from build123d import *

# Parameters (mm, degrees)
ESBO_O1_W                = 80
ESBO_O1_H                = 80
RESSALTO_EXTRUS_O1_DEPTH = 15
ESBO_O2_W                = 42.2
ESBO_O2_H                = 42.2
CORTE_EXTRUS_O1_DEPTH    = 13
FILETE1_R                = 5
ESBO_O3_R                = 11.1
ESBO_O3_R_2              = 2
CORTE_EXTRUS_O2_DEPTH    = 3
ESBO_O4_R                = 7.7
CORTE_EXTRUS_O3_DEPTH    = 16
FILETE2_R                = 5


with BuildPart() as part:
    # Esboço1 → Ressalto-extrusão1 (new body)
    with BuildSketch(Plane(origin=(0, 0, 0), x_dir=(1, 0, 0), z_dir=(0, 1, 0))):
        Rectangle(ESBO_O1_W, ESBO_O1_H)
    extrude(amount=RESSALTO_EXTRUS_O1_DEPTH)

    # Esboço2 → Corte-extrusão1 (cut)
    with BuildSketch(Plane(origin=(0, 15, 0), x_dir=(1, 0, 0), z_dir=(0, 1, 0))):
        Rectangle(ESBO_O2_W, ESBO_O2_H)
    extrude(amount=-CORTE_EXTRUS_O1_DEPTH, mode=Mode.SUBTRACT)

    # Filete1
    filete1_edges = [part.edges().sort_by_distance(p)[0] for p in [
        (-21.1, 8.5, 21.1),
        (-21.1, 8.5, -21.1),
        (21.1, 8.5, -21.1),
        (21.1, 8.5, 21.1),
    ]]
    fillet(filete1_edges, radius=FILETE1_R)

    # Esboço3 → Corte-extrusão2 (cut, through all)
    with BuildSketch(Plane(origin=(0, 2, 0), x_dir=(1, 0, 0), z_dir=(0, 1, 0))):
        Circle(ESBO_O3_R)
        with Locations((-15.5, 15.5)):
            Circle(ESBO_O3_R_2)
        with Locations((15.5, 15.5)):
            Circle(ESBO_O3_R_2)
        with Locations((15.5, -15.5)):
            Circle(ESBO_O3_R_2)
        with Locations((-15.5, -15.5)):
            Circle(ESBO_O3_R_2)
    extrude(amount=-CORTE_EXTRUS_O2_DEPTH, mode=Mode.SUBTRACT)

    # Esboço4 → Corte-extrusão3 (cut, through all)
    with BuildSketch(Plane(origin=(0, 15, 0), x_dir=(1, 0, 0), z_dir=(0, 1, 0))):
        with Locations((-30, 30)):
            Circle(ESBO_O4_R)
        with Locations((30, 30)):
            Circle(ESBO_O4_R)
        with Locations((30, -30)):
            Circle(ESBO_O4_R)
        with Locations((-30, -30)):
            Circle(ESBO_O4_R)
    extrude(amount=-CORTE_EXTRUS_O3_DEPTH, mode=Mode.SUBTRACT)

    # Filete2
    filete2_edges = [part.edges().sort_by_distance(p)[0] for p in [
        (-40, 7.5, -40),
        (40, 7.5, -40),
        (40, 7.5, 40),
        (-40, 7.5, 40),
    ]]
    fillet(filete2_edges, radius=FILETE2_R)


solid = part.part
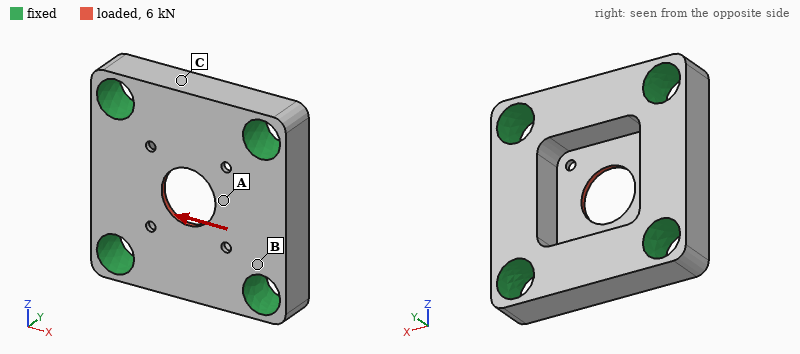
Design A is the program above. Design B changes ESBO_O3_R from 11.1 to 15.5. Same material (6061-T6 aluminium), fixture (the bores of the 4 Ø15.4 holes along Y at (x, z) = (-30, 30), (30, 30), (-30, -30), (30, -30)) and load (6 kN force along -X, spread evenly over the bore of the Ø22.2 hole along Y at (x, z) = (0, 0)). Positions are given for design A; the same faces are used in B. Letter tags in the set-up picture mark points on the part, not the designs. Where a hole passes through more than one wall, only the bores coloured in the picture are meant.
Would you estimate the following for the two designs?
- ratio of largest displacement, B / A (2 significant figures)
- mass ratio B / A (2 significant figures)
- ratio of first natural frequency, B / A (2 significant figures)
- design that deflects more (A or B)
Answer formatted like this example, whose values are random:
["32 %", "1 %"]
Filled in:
["0.82", "0.99", "1.6", "A"]
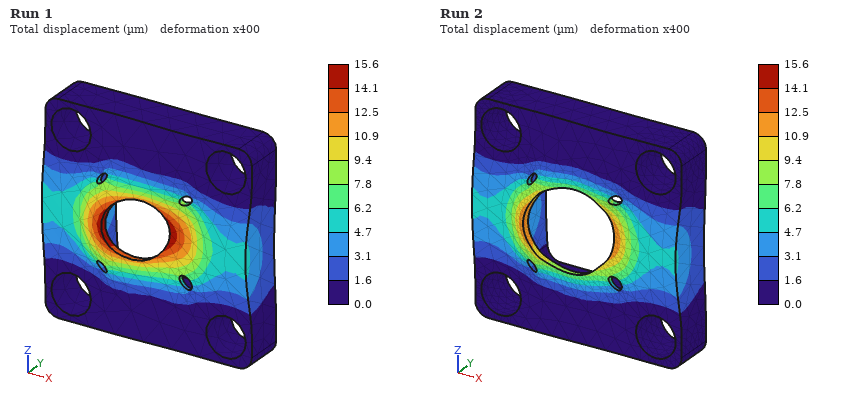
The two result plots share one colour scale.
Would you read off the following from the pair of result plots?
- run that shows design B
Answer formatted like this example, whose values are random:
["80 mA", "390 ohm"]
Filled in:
["Run 2"]
